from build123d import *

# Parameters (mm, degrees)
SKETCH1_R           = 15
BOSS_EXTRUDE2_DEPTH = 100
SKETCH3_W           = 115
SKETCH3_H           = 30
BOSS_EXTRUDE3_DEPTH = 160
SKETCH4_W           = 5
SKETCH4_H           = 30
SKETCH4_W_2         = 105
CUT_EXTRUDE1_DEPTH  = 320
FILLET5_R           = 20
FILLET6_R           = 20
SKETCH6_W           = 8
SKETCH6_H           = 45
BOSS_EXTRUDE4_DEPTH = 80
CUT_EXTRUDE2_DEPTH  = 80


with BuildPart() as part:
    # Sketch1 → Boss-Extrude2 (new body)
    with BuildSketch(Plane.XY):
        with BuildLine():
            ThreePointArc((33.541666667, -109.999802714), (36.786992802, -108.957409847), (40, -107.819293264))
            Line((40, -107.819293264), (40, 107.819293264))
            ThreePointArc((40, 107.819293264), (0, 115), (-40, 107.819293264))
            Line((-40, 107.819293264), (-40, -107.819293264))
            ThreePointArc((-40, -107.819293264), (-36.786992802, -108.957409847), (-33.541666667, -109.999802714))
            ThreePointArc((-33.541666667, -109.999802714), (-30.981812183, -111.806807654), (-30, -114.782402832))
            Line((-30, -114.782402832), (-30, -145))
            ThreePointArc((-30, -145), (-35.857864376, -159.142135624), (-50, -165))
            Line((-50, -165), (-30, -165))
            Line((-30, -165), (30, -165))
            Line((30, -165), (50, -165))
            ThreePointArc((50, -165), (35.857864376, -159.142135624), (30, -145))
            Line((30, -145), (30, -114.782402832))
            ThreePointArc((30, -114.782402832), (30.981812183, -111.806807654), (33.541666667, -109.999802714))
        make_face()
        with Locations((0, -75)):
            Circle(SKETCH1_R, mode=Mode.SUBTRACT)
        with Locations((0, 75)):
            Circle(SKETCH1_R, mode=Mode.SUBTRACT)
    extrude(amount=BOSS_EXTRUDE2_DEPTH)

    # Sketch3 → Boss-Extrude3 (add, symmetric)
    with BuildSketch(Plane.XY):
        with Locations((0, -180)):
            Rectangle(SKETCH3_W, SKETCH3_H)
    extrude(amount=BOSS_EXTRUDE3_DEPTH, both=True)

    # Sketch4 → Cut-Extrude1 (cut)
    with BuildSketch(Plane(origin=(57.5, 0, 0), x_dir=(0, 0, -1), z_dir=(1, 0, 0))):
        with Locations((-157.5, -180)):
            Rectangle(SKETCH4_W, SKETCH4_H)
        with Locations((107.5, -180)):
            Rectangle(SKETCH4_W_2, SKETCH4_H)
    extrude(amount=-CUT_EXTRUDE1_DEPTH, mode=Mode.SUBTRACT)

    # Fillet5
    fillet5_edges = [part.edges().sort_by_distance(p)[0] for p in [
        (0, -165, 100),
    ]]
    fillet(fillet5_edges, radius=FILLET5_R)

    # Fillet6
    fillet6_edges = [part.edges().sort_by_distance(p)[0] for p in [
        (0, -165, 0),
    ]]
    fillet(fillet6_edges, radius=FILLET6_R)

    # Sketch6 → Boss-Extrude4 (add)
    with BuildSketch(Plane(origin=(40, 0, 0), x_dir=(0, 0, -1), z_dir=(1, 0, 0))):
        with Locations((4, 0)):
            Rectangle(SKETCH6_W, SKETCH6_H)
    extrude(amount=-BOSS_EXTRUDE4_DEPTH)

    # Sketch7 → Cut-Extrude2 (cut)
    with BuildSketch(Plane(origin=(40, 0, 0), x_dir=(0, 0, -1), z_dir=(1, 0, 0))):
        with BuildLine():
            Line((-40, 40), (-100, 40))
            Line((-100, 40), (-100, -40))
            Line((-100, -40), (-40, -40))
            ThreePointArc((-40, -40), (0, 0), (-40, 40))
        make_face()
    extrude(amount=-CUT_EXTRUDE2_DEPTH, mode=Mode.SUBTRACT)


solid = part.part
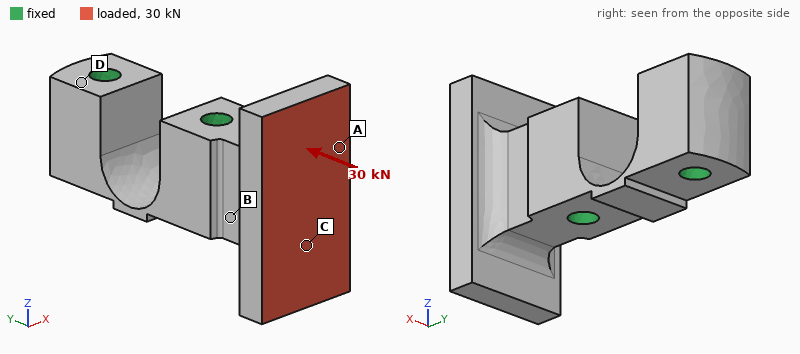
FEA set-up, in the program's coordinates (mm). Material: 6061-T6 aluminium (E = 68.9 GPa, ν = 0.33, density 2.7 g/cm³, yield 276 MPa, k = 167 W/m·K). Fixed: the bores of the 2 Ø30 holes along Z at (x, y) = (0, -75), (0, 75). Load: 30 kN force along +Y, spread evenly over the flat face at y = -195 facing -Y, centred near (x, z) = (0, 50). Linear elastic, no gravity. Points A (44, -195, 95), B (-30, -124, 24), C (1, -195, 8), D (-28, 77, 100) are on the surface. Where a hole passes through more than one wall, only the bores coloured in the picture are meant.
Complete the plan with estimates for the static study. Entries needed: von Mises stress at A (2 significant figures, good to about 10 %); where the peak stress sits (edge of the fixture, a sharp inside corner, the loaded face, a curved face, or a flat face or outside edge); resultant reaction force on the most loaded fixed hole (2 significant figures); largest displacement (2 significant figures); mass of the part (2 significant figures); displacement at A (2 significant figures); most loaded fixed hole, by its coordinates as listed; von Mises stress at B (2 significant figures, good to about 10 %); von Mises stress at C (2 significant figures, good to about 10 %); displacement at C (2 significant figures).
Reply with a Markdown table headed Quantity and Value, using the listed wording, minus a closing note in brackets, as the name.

| Quantity | Value |
|---|---|
| von Mises stress at A | 7.5 MPa |
| where the peak stress sits | a curved face |
| resultant reaction force on the most loaded fixed hole | 30 kN |
| largest displacement | 30 µm |
| mass of the part | 5.9 kg |
| displacement at A | 10 µm |
| most loaded fixed hole, by its coordinates as listed | (0, -75) |
| von Mises stress at B | 5.0 MPa |
| von Mises stress at C | 8.5 MPa |
| displacement at C | 8.5 µm |
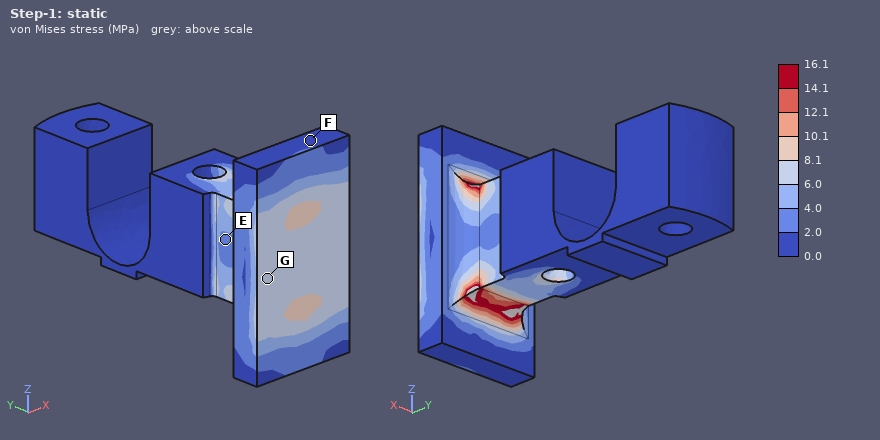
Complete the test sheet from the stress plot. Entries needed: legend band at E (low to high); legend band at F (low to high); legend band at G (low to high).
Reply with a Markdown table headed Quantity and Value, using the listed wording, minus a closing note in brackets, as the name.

| Quantity | Value |
|---|---|
| legend band at E | 2.0 to 4.0 MPa |
| legend band at F | 0.0 to 2.0 MPa |
| legend band at G | 6.0 to 8.1 MPa |
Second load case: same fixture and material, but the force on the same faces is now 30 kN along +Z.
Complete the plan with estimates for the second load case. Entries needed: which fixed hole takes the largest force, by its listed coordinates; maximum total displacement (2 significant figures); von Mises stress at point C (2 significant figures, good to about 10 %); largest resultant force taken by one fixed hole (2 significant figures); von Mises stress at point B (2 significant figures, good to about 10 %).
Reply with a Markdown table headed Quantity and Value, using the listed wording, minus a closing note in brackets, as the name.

| Quantity | Value |
|---|---|
| which fixed hole takes the largest force, by its listed coordinates | (0, -75) |
| maximum total displacement | 96 µm |
| von Mises stress at point C | 8.3 MPa |
| largest resultant force taken by one fixed hole | 30 kN |
| von Mises stress at point B | 15 MPa |
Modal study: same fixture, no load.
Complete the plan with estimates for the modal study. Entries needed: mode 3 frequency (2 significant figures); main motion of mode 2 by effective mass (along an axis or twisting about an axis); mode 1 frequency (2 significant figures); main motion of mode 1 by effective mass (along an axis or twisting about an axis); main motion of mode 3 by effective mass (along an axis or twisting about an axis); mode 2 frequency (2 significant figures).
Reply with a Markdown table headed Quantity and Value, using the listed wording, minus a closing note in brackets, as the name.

| Quantity | Value |
|---|---|
| mode 3 frequency | 2300 Hz |
| main motion of mode 2 by effective mass | twisting about Y |
| mode 1 frequency | 1700 Hz |
| main motion of mode 1 by effective mass | along X |
| main motion of mode 3 by effective mass | along Z |
| mode 2 frequency | 2100 Hz |
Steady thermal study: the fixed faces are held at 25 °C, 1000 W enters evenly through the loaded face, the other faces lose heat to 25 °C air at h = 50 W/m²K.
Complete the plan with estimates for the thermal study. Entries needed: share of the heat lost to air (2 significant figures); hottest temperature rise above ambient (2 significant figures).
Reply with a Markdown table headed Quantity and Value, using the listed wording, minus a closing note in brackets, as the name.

| Quantity | Value |
|---|---|
| share of the heat lost to air | 18 % |
| hottest temperature rise above ambient | 85 K |
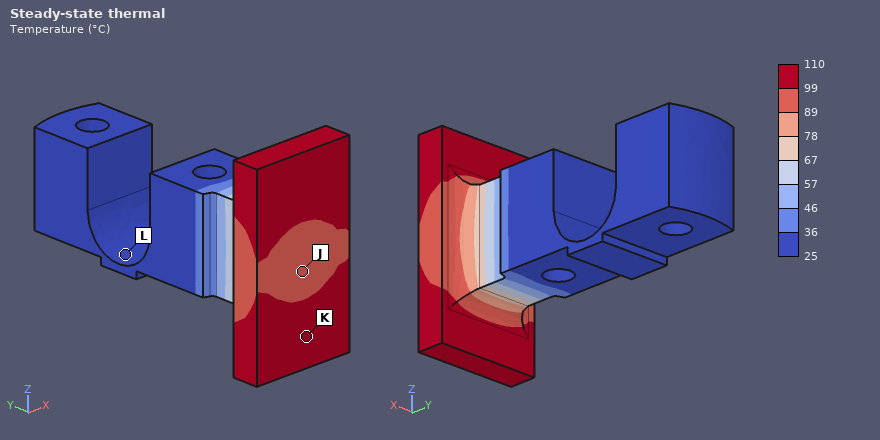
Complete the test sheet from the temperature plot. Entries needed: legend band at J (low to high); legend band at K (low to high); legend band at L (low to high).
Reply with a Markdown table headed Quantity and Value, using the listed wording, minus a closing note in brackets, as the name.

| Quantity | Value |
|---|---|
| legend band at J | 89 to 99 °C |
| legend band at K | 99 to 110 °C |
| legend band at L | 25 to 36 °C |
